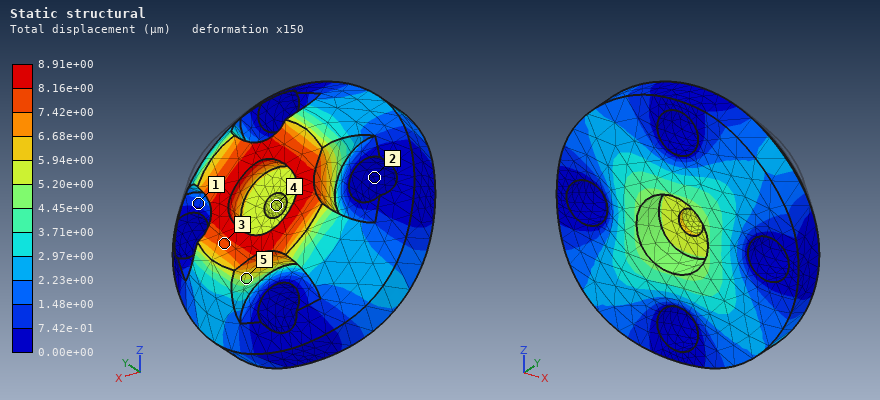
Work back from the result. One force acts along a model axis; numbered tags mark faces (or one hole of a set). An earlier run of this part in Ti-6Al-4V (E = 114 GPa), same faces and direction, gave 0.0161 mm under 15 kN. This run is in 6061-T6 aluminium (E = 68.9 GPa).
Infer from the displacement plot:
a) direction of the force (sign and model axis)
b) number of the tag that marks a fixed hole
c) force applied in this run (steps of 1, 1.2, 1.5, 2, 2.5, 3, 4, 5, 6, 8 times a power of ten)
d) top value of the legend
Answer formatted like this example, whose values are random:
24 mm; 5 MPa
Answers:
-Y; 2; 5 kN; 8.91e+00 µm
